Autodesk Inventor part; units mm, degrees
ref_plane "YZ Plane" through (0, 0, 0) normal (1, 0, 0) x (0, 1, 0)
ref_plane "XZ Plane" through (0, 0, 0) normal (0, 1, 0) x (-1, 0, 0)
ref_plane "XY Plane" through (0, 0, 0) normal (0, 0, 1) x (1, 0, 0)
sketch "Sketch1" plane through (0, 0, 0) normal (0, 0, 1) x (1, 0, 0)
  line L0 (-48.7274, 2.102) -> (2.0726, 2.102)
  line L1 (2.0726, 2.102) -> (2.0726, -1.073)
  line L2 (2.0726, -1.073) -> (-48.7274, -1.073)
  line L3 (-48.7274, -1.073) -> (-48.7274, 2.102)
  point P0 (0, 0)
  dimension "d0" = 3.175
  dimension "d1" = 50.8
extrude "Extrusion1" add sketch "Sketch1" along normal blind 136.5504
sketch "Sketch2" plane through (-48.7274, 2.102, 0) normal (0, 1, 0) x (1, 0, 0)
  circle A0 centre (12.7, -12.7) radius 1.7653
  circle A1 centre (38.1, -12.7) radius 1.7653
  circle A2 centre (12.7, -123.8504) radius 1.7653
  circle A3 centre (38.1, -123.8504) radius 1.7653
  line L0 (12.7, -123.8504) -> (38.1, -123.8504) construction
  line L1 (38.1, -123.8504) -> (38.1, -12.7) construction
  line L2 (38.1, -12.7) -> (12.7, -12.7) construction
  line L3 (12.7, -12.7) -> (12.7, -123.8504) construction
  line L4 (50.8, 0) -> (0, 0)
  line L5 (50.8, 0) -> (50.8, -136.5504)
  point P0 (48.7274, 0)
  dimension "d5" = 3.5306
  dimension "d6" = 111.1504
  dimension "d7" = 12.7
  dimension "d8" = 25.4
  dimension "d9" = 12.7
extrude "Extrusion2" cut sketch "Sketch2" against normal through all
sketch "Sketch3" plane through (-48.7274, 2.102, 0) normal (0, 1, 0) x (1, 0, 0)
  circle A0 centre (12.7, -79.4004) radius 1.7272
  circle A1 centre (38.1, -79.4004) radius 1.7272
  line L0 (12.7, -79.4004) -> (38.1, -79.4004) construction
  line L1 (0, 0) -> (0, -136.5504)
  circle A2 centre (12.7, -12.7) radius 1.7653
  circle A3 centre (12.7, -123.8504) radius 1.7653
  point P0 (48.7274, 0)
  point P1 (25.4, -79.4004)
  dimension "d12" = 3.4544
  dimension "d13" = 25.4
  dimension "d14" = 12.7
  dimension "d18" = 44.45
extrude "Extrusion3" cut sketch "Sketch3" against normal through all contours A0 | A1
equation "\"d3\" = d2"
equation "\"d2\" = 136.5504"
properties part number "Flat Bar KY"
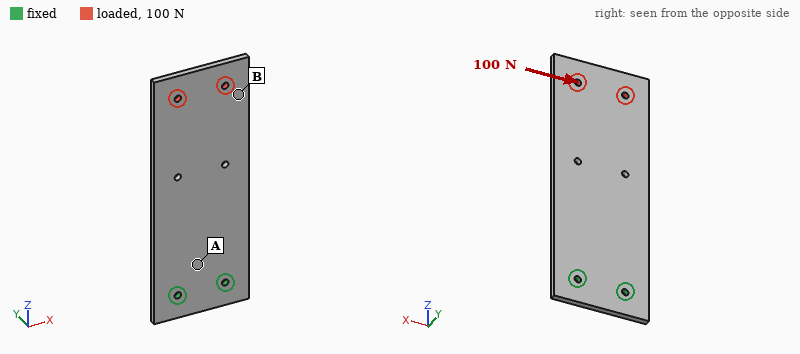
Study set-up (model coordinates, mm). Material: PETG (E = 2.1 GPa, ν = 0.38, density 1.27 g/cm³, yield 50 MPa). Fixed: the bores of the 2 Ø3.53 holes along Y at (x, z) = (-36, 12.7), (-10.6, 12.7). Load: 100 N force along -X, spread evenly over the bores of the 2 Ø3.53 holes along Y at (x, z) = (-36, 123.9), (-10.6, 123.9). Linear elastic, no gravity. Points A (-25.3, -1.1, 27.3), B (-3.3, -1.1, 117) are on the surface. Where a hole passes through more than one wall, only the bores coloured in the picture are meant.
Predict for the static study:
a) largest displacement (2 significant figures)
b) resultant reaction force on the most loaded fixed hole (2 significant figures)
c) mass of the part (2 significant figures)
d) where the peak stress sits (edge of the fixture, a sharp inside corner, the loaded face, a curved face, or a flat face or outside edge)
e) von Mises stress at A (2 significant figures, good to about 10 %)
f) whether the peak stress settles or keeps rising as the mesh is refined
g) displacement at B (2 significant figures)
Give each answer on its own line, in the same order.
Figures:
1.2 mm
410 N
28 g
edge of the fixture
3.1 MPa
keeps rising
0.94 mm
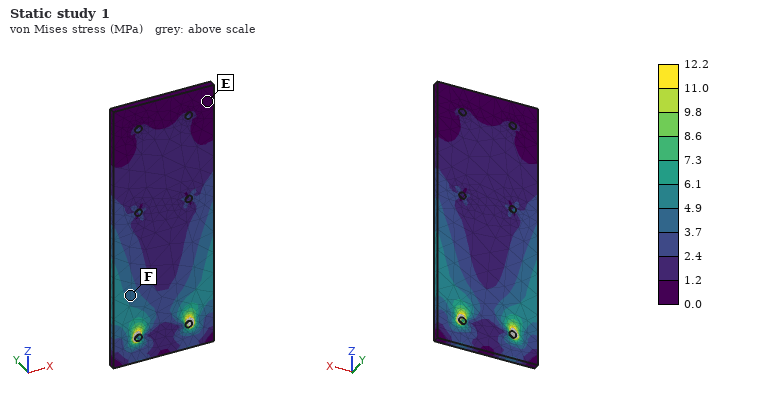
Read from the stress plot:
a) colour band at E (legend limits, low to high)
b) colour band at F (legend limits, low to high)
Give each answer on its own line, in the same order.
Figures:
0.0 to 1.2 MPa
3.7 to 4.9 MPa
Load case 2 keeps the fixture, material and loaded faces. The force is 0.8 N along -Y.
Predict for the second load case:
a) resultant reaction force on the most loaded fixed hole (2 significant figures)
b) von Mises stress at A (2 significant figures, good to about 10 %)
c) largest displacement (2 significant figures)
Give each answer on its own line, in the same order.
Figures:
0.40 N
0.83 MPa
1.5 mm
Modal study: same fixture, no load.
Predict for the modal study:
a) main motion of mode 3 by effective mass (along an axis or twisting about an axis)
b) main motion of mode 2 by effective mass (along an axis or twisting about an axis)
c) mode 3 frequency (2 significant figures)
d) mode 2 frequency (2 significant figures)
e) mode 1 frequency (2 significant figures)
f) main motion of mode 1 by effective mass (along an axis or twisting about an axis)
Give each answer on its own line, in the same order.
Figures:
along Y
twisting about Z
270 Hz
210 Hz
44 Hz
along Y
